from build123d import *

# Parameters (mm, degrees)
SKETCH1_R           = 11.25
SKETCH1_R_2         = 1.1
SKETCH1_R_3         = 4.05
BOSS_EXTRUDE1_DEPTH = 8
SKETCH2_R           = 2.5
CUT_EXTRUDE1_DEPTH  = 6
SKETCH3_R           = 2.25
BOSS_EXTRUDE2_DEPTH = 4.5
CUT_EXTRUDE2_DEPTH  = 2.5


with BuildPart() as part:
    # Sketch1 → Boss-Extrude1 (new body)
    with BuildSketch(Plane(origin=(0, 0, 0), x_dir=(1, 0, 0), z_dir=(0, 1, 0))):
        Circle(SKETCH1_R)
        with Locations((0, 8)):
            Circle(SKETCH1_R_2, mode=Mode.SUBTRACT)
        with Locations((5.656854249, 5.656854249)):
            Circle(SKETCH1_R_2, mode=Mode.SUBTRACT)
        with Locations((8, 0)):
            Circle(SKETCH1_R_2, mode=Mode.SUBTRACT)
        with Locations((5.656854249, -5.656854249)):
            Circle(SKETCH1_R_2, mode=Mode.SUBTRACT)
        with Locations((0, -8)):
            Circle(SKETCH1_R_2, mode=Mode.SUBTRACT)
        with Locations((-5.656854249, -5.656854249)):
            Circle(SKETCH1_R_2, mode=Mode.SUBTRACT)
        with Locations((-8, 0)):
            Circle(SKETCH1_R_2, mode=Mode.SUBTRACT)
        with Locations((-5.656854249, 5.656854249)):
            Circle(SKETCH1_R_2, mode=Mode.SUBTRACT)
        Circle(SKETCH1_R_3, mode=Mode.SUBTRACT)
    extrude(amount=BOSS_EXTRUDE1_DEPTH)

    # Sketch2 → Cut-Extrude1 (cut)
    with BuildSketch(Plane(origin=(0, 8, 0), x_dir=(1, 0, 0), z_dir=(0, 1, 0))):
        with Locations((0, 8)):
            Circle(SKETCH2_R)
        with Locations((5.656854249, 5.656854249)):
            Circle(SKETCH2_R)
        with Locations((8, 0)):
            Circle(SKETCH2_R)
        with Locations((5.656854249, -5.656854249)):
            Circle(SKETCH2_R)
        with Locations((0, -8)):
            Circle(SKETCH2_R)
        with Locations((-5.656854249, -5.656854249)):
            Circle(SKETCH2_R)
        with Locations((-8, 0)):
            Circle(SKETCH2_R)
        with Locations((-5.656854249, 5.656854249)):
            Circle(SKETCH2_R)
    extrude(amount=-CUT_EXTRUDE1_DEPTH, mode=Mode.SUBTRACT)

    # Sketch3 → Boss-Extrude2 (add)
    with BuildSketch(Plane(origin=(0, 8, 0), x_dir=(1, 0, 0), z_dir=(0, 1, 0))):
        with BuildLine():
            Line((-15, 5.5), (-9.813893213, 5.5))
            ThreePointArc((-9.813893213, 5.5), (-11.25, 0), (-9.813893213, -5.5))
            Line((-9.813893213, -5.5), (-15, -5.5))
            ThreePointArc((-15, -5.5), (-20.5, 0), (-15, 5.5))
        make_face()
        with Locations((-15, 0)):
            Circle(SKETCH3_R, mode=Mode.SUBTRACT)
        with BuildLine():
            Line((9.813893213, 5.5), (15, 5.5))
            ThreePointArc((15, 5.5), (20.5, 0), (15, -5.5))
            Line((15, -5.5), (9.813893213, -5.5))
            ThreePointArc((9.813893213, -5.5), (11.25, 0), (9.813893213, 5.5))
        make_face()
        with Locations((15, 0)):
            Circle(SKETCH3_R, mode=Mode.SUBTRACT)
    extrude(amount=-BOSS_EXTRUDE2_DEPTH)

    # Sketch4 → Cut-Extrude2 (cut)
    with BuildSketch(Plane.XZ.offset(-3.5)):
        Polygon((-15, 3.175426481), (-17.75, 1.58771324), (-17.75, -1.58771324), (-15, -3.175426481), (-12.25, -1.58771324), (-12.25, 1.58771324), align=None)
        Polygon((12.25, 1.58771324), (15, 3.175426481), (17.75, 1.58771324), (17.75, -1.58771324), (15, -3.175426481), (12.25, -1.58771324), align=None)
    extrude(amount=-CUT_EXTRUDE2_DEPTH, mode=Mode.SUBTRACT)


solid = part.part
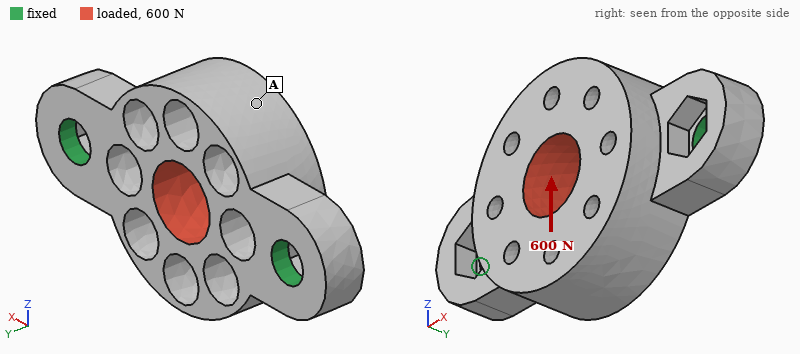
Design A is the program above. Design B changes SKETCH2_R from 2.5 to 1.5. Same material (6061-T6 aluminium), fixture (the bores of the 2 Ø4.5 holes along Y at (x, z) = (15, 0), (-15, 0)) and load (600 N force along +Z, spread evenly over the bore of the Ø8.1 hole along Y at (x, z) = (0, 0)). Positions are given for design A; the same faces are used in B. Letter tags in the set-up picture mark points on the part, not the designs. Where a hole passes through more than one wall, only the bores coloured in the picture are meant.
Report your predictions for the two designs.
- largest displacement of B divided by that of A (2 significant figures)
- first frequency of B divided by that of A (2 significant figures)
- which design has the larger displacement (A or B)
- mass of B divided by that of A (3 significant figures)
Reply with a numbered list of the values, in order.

1. 0.90
2. 0.94
3. A
4. 1.25
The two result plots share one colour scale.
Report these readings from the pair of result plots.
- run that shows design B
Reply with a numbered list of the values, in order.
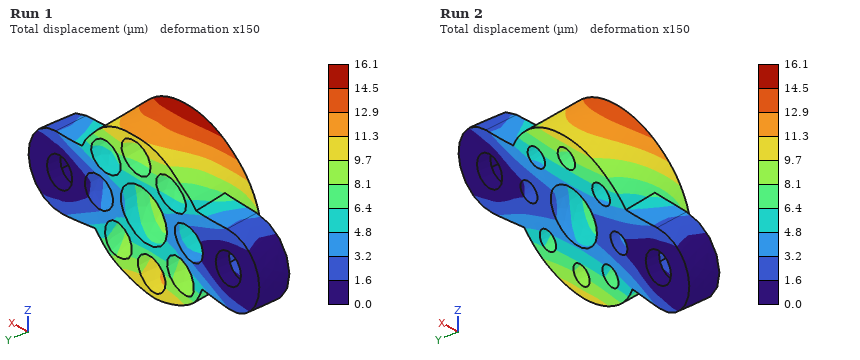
1. Run 2
